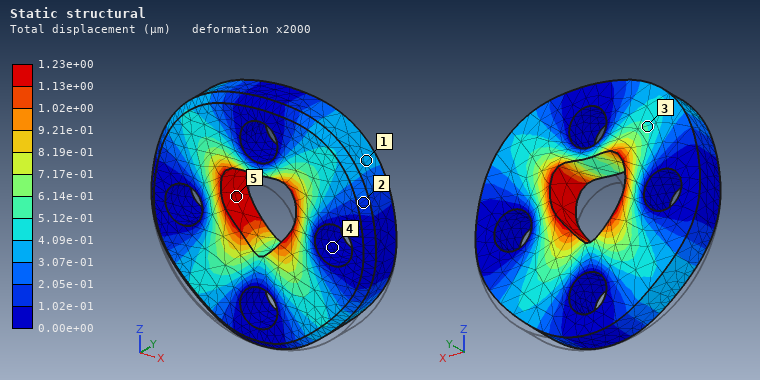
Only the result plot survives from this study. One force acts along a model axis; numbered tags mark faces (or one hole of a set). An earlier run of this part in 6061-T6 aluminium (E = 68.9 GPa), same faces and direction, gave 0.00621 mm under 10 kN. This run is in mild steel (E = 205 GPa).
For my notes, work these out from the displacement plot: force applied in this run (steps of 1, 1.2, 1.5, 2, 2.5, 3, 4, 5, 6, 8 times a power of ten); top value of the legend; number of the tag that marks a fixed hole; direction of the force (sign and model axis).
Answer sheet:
6 kN
1.23e+00 µm
4
+Z
